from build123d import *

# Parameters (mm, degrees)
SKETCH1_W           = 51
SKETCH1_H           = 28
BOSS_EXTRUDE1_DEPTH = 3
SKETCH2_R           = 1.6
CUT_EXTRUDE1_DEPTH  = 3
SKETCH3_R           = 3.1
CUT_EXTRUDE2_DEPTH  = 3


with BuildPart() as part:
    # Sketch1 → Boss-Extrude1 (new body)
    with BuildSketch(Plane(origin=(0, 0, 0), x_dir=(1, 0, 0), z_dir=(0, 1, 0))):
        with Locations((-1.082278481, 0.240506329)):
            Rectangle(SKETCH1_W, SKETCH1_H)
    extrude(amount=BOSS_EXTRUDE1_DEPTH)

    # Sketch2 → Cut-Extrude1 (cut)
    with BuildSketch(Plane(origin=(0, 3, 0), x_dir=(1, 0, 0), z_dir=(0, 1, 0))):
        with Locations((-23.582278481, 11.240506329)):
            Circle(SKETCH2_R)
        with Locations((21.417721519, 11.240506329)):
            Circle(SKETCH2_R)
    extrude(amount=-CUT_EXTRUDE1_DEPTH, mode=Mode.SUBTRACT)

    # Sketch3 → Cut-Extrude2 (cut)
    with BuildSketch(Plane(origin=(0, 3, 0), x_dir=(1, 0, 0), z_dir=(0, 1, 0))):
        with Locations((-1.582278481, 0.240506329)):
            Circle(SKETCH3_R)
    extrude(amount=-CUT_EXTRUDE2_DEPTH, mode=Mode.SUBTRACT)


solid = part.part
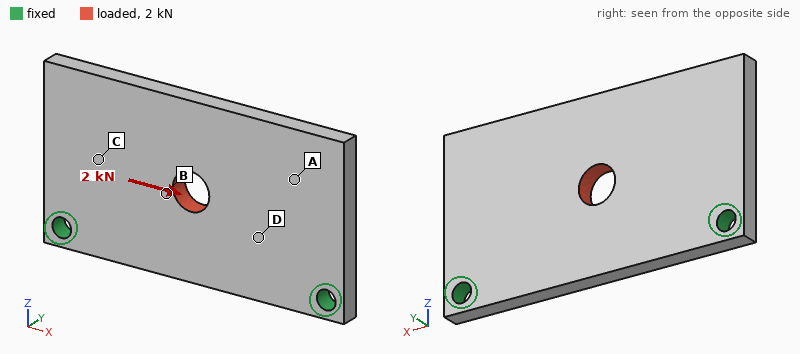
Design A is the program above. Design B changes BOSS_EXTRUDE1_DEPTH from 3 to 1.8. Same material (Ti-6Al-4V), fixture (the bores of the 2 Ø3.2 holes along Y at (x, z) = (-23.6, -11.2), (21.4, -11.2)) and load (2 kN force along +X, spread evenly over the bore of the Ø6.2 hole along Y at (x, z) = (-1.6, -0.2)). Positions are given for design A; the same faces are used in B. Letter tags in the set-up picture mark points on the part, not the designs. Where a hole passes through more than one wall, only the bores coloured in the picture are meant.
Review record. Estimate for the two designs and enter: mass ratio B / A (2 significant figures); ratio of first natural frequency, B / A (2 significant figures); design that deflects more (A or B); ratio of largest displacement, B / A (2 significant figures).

0.60
0.63
B
1.7
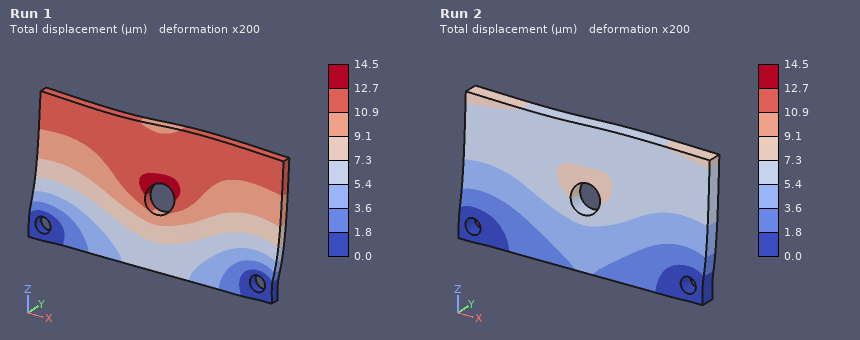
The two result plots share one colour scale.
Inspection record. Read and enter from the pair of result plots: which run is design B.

Run 1
